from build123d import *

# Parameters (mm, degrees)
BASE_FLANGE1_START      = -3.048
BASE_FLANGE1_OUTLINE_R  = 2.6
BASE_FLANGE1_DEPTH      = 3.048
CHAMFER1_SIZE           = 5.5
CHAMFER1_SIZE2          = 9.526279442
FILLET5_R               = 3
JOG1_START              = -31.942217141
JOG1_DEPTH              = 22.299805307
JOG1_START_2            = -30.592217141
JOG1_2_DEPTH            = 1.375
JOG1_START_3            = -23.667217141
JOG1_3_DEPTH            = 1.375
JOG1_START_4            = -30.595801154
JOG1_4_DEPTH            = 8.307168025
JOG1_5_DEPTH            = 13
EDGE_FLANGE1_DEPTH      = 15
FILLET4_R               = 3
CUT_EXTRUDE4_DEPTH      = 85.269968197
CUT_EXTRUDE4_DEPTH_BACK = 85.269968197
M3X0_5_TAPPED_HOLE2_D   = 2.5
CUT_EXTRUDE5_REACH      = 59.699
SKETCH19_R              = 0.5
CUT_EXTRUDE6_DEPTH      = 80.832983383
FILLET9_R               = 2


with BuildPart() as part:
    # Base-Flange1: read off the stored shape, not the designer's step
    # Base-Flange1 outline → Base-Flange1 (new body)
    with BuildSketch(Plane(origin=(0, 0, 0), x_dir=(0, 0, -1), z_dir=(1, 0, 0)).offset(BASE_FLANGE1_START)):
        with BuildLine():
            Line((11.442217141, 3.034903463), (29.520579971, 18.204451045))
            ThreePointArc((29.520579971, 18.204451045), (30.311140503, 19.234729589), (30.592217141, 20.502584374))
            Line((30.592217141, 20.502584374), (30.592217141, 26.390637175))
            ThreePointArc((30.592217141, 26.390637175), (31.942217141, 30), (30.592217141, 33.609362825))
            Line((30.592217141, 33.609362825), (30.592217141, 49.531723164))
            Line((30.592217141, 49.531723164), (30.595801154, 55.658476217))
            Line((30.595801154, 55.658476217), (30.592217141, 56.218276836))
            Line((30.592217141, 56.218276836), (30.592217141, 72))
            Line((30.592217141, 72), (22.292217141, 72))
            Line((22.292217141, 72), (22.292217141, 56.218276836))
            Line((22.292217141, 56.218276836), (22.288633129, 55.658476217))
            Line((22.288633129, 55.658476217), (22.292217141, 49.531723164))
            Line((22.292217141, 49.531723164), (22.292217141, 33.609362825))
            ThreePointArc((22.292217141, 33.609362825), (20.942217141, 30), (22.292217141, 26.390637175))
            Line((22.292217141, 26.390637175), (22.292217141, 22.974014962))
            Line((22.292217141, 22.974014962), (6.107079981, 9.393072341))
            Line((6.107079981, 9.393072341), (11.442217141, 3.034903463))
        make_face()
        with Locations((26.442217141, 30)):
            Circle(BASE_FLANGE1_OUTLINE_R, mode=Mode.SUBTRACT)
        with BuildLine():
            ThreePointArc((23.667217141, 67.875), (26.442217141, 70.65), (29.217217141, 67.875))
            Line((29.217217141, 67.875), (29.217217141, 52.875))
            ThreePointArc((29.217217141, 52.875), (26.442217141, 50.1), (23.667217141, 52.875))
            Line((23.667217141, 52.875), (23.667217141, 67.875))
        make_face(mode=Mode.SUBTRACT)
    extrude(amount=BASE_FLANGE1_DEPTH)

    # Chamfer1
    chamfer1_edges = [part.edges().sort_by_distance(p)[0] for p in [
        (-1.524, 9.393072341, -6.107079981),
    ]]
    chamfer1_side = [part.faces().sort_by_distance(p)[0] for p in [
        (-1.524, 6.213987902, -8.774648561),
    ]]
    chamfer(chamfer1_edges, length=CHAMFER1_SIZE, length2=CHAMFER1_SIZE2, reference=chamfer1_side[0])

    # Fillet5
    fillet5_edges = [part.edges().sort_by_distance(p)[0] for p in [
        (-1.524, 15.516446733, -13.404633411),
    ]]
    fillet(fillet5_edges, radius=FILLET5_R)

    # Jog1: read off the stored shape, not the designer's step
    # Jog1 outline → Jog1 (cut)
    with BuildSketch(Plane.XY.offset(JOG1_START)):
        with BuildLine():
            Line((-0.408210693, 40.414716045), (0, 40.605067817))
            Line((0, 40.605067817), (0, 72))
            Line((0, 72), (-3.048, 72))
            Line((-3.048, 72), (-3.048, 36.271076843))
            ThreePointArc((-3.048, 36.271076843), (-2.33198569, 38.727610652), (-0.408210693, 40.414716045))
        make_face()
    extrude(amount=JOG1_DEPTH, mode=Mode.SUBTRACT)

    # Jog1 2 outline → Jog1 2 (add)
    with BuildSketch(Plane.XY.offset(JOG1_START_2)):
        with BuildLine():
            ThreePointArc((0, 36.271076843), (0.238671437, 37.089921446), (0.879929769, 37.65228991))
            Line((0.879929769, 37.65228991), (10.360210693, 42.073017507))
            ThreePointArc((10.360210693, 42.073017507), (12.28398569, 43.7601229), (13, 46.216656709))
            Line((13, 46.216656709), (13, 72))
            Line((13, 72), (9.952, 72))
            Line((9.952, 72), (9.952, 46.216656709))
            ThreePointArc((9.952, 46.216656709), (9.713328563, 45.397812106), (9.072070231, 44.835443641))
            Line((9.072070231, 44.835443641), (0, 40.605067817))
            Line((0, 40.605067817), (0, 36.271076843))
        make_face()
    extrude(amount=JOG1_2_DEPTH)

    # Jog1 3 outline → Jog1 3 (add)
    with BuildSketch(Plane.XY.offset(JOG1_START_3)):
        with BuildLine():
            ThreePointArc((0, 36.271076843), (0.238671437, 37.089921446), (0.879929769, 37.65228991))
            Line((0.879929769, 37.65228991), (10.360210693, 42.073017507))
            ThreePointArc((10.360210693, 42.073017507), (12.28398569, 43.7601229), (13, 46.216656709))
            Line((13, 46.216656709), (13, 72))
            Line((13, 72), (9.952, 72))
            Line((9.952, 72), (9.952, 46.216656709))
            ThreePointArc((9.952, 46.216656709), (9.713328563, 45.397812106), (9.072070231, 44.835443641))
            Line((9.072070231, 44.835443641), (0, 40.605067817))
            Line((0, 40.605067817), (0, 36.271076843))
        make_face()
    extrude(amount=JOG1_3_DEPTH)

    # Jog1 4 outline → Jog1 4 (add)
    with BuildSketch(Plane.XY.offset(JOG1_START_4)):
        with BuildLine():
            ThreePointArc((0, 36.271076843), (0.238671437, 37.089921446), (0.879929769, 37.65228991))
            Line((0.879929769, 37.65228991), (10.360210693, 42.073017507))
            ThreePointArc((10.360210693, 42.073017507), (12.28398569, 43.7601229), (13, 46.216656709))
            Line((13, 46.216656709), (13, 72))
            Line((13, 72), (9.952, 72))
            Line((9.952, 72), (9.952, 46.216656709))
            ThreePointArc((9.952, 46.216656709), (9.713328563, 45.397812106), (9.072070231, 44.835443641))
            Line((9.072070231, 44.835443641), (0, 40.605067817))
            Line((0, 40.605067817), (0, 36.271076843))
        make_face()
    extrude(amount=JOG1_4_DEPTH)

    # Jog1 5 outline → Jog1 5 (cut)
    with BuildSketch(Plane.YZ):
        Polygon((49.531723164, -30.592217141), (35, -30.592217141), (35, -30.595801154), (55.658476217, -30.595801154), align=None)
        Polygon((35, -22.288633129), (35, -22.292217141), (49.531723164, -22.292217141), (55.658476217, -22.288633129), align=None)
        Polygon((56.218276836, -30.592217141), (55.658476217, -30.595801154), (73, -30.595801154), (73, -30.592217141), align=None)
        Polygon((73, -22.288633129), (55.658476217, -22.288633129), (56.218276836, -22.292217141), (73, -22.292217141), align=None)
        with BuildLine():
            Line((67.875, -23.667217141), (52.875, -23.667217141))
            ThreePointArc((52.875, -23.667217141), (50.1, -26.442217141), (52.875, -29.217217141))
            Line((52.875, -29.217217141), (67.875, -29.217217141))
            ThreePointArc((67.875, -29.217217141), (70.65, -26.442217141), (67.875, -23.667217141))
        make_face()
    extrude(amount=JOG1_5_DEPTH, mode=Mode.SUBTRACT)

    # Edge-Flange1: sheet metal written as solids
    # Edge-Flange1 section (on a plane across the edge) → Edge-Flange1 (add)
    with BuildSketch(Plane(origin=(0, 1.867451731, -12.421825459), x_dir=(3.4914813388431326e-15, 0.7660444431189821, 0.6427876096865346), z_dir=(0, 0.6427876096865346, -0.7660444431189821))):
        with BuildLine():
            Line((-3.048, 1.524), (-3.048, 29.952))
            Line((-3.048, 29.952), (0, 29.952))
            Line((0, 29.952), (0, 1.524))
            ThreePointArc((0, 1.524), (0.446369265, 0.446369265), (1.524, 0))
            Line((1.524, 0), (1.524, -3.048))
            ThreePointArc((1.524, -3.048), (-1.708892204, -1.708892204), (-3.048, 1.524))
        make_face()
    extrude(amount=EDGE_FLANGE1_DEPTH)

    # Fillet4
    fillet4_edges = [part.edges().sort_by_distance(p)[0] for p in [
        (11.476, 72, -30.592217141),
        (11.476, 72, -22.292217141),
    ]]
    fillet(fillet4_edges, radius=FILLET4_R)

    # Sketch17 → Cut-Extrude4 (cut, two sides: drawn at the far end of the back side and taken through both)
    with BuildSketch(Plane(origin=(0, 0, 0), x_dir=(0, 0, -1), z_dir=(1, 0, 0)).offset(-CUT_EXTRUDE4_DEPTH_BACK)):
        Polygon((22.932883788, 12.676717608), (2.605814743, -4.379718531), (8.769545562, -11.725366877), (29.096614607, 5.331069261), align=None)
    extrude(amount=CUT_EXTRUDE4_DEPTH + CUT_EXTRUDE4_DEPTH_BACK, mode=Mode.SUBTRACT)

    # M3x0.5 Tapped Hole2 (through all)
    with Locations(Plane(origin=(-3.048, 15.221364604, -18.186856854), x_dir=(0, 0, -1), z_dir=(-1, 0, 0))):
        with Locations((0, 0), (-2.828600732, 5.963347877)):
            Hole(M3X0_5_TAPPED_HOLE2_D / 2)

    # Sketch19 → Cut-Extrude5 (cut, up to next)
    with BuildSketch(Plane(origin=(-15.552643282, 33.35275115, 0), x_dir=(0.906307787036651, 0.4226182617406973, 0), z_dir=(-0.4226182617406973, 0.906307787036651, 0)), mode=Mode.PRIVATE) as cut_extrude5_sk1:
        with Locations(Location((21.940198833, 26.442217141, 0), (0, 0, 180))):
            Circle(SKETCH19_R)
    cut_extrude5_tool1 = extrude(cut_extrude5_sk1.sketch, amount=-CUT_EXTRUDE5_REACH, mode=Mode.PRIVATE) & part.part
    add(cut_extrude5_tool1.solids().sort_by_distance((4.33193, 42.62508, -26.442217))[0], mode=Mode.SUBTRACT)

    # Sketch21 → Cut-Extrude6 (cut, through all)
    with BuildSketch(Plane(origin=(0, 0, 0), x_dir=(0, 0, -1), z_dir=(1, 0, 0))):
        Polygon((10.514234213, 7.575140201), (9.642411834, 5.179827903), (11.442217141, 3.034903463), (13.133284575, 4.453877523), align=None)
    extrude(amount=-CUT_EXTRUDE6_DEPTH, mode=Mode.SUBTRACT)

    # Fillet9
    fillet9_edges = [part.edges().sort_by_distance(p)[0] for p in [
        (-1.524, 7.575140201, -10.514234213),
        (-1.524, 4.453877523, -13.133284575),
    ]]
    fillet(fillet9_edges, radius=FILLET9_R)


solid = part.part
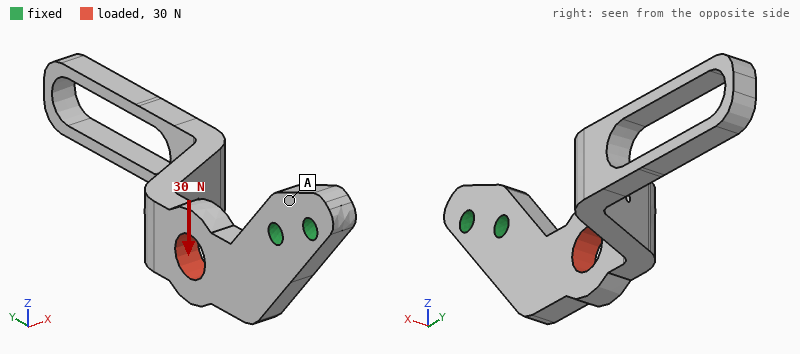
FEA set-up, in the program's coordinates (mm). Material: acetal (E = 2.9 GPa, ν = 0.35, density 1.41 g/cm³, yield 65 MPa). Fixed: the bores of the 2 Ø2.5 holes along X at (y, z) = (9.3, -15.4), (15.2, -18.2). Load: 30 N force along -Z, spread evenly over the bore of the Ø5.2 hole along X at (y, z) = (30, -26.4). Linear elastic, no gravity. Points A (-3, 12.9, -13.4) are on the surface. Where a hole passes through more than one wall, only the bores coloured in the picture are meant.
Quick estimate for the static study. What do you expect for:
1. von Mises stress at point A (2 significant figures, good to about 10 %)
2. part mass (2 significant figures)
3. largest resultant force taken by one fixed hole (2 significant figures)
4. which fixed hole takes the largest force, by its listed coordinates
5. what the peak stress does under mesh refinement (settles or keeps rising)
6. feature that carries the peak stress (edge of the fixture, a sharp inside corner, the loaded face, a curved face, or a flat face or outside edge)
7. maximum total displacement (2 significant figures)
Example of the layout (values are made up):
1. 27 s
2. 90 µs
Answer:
1. 1.7 MPa
2. 2.2 g
3. 71 N
4. (15.2, -18.2)
5. keeps rising
6. edge of the fixture
7. 0.76 mm
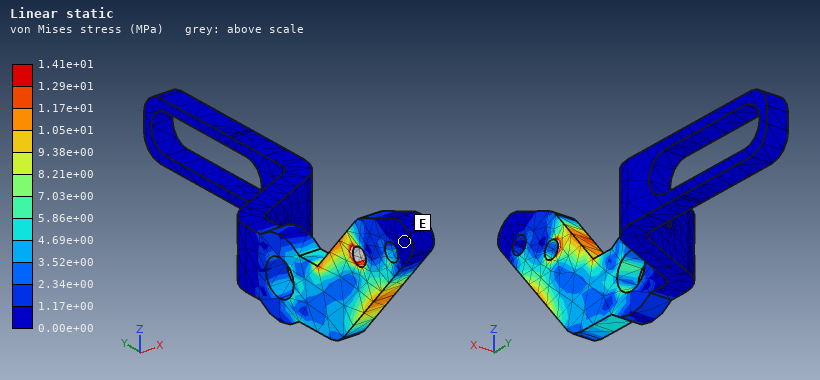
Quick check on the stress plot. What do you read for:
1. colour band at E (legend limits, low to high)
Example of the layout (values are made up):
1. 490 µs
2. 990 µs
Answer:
1. 0.00e+00 to 1.17e+00 MPa
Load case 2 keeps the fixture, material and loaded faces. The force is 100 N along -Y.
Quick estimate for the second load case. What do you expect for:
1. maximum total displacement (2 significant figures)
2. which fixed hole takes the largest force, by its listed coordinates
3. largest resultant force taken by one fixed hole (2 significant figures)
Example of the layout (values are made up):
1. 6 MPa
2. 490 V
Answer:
1. 0.85 mm
2. (15.2, -18.2)
3. 120 N
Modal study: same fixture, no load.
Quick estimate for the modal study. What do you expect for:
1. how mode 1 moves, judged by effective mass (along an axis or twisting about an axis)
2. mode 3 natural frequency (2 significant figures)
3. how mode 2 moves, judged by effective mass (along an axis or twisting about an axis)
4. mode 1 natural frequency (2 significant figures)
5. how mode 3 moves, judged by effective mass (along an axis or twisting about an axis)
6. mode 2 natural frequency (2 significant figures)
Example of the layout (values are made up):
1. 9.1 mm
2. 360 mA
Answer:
1. along X
2. 1000 Hz
3. along Z
4. 240 Hz
5. along X
6. 460 Hz
